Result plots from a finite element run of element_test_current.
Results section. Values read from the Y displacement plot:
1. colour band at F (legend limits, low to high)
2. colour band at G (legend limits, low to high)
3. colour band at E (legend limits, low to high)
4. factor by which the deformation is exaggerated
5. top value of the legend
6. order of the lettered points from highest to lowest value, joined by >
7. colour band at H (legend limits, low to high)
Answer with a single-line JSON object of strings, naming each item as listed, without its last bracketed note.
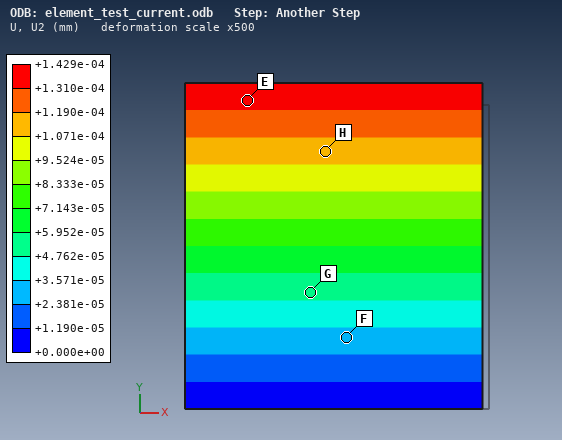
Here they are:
{"colour band at F": "+2.381e-05 to +3.571e-05 mm", "colour band at G": "+4.762e-05 to +5.952e-05 mm", "colour band at E": "+1.310e-04 to +1.429e-04 mm", "factor by which the deformation is exaggerated": "500", "top value of the legend": "+1.429e-04 mm", "order of the lettered points from highest to lowest value, joined by >": "E > H > G > F", "colour band at H": "+1.071e-04 to +1.190e-04 mm"}
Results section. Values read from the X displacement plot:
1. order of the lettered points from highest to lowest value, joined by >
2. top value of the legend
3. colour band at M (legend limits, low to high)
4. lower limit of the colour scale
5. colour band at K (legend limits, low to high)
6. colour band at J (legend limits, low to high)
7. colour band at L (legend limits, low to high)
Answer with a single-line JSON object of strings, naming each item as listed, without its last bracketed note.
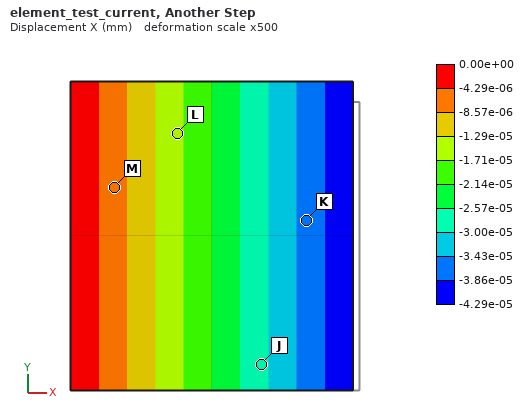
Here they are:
{"order of the lettered points from highest to lowest value, joined by >": "M > L > J > K", "top value of the legend": "0.00e+00 mm", "colour band at M": "-8.57e-06 to -4.29e-06 mm", "lower limit of the colour scale": "-4.29e-05 mm", "colour band at K": "-3.86e-05 to -3.43e-05 mm", "colour band at J": "-3.00e-05 to -2.57e-05 mm", "colour band at L": "-1.71e-05 to -1.29e-05 mm"}
